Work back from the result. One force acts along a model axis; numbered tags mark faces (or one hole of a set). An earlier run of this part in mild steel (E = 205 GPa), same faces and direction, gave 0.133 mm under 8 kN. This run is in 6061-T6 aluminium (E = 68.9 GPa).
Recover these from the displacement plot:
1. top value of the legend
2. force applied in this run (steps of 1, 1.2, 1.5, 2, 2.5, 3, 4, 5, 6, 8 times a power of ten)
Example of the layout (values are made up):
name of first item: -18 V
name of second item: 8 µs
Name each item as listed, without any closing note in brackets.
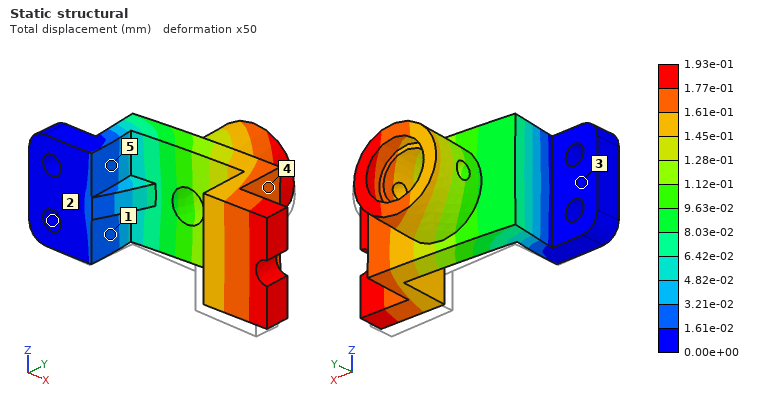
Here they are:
top value of the legend: 1.93e-01 mm
force applied in this run: 4 kN
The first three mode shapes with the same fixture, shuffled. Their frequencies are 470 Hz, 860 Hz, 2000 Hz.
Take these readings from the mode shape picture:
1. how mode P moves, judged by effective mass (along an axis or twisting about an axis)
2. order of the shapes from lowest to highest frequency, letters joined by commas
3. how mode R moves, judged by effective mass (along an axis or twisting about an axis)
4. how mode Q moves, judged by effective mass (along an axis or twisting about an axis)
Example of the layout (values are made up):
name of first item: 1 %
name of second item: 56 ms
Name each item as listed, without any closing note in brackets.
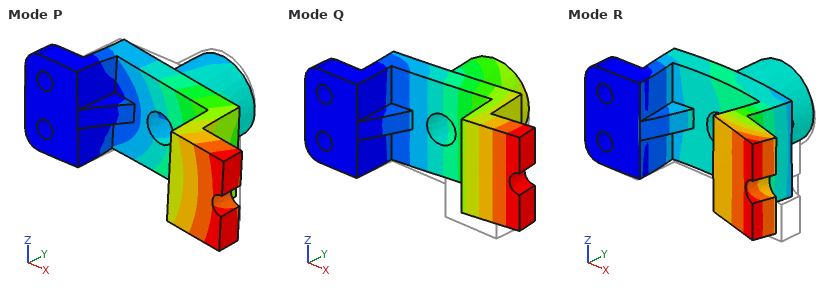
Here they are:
how mode P moves, judged by effective mass: along Z
order of the shapes from lowest to highest frequency, letters joined by commas: Q, P, R
how mode R moves, judged by effective mass: along X
how mode Q moves, judged by effective mass: along Y
